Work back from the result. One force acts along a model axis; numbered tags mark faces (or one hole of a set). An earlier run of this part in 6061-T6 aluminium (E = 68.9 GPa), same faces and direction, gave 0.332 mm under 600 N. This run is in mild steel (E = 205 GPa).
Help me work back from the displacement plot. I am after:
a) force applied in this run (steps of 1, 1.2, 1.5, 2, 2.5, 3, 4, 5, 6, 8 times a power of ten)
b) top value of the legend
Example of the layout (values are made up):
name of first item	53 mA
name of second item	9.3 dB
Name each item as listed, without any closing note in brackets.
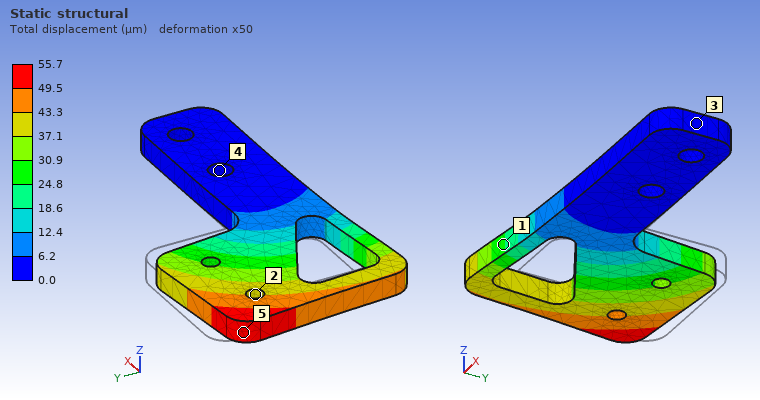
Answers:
force applied in this run	300 N
top value of the legend	55.7 µm
